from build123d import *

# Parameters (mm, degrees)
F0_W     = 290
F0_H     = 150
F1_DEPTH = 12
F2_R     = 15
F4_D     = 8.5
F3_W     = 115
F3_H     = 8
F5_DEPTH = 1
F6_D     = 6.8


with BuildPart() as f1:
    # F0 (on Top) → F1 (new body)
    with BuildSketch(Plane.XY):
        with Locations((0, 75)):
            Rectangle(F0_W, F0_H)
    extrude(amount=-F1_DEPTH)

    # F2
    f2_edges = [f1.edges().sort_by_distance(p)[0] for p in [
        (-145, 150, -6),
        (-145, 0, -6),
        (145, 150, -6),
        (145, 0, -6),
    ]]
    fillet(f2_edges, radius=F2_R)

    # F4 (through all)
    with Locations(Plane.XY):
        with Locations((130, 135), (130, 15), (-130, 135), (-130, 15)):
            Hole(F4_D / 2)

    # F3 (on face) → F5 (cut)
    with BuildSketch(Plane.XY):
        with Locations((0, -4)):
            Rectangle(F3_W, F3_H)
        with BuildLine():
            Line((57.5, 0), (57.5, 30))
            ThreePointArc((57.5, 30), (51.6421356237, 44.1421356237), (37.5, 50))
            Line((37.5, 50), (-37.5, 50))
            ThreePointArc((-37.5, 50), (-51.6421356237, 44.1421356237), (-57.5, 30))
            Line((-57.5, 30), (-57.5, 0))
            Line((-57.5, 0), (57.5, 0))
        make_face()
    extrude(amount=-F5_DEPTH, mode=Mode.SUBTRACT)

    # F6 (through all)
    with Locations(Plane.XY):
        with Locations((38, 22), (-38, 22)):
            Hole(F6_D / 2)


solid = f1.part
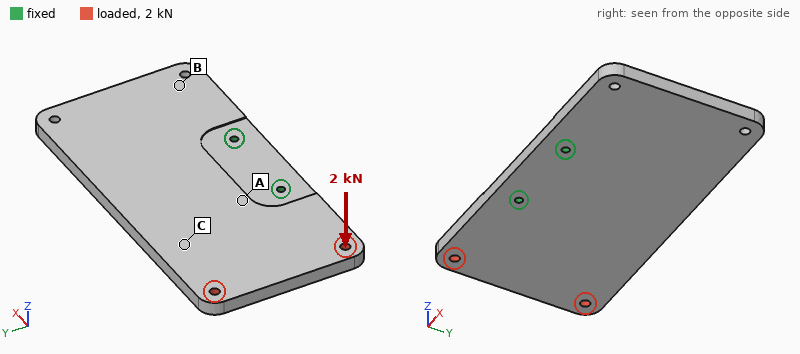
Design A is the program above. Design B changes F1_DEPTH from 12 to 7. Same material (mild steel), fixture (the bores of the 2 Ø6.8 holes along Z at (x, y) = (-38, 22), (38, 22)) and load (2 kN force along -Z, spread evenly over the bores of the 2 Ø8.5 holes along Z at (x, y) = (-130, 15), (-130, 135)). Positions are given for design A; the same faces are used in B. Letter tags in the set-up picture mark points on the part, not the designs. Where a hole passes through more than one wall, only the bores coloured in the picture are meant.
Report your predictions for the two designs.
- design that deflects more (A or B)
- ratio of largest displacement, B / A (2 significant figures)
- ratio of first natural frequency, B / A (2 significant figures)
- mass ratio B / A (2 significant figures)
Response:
B
5.1
0.58
0.58
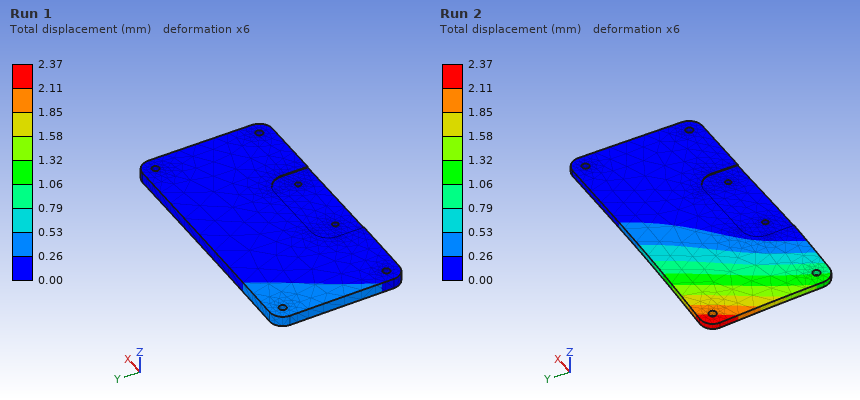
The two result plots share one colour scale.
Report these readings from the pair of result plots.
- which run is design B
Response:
Run 2
